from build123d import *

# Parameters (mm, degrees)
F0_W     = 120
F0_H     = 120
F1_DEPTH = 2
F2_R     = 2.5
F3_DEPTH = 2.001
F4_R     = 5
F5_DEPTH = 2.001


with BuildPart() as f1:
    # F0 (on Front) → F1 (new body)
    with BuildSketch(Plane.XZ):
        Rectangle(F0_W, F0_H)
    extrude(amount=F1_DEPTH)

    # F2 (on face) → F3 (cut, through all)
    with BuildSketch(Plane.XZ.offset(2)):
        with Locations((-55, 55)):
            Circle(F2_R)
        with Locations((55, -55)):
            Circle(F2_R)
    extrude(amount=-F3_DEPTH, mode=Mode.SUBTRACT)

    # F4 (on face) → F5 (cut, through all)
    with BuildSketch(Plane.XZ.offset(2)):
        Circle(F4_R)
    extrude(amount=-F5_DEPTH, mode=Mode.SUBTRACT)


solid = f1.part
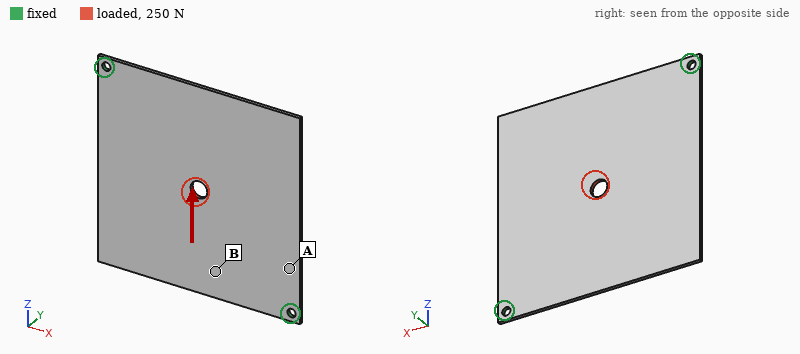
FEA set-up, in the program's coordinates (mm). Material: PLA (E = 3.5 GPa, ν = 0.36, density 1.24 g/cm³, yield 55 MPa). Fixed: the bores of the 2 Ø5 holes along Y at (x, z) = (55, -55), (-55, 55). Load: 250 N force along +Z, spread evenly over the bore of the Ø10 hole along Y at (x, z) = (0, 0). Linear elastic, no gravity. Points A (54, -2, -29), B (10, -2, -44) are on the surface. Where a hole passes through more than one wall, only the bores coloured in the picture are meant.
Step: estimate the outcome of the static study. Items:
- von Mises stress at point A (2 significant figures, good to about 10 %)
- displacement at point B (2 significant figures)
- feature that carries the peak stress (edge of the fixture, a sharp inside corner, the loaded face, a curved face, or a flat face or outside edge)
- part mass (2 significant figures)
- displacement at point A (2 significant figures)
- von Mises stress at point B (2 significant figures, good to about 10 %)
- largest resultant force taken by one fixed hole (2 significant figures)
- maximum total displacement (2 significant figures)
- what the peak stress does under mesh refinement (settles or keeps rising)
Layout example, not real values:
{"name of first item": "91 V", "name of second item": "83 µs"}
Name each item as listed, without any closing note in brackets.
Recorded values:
{"von Mises stress at point A": "2.7 MPa", "displacement at point B": "65 µm", "feature that carries the peak stress": "edge of the fixture", "part mass": "35 g", "displacement at point A": "35 µm", "von Mises stress at point B": "0.91 MPa", "largest resultant force taken by one fixed hole": "130 N", "maximum total displacement": "86 µm", "what the peak stress does under mesh refinement": "keeps rising"}
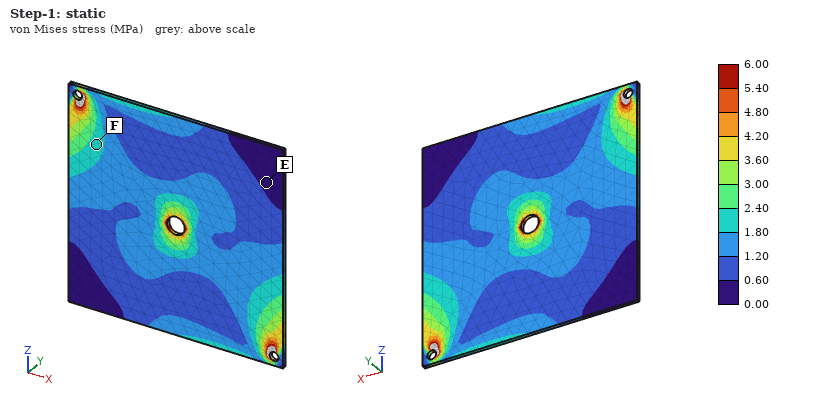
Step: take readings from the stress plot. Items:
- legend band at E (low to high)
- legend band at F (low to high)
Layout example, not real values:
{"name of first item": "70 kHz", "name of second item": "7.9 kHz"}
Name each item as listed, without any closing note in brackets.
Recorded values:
{"legend band at E": "0.00 to 0.60 MPa", "legend band at F": "1.80 to 2.40 MPa"}
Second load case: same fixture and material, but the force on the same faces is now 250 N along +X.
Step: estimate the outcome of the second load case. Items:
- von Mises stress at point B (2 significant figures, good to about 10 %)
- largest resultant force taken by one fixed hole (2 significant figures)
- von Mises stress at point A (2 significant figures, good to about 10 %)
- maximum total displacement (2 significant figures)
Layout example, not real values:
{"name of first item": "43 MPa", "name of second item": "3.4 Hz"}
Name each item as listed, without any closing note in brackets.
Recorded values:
{"von Mises stress at point B": "1.5 MPa", "largest resultant force taken by one fixed hole": "130 N", "von Mises stress at point A": "1.3 MPa", "maximum total displacement": "86 µm"}
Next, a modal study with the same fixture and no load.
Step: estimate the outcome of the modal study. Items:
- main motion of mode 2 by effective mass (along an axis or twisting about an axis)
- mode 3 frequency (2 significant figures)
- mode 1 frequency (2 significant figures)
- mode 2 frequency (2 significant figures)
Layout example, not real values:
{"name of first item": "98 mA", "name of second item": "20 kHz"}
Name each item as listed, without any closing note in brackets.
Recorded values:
{"main motion of mode 2 by effective mass": "along Y", "mode 3 frequency": "240 Hz", "mode 1 frequency": "59 Hz", "mode 2 frequency": "81 Hz"}
